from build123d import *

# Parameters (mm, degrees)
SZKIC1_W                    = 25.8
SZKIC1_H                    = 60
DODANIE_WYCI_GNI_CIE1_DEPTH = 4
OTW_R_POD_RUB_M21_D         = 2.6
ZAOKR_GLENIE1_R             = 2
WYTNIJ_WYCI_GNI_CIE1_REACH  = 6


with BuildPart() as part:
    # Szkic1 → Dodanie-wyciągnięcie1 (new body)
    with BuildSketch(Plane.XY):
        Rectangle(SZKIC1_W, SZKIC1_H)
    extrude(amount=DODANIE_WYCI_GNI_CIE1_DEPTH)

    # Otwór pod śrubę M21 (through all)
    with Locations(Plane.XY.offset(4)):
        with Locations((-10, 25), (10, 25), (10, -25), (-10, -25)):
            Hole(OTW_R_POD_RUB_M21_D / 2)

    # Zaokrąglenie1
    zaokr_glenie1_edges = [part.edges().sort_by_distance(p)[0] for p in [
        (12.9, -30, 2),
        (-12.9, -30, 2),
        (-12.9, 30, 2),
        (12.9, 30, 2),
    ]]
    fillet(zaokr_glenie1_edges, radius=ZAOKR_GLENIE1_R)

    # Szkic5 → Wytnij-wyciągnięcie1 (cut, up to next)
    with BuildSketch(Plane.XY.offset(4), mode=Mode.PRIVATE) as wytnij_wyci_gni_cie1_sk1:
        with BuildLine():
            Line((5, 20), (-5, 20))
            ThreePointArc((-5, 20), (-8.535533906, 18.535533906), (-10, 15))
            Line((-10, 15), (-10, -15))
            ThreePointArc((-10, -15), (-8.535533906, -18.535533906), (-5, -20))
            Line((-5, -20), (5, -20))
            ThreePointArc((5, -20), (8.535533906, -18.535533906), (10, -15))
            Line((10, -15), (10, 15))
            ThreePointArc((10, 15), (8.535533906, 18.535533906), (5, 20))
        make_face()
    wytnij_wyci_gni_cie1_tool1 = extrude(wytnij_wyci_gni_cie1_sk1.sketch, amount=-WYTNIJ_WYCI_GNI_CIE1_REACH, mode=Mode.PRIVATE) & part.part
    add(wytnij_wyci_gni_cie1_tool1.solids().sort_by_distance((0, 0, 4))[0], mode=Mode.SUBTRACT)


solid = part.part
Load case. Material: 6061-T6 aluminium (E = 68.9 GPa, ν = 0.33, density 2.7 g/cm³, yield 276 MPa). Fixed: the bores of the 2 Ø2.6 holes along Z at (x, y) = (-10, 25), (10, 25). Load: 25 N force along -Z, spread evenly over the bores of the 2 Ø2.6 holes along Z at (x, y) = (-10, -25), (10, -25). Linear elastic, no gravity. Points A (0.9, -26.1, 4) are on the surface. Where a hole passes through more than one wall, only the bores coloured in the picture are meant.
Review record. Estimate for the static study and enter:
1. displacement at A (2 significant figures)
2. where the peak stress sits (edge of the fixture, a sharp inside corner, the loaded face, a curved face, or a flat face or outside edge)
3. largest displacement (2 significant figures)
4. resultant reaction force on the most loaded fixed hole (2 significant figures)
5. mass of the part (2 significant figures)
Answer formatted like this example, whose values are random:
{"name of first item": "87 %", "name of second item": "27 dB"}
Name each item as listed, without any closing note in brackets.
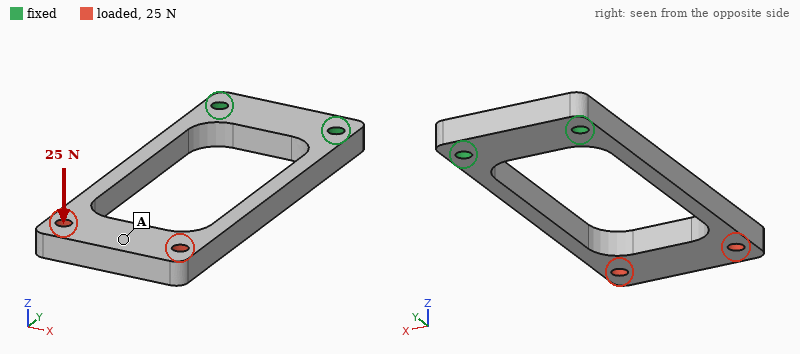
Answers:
{"displacement at A": "0.41 mm", "where the peak stress sits": "a curved face", "largest displacement": "0.46 mm", "resultant reaction force on the most loaded fixed hole": "13 N", "mass of the part": "8.0 g"}
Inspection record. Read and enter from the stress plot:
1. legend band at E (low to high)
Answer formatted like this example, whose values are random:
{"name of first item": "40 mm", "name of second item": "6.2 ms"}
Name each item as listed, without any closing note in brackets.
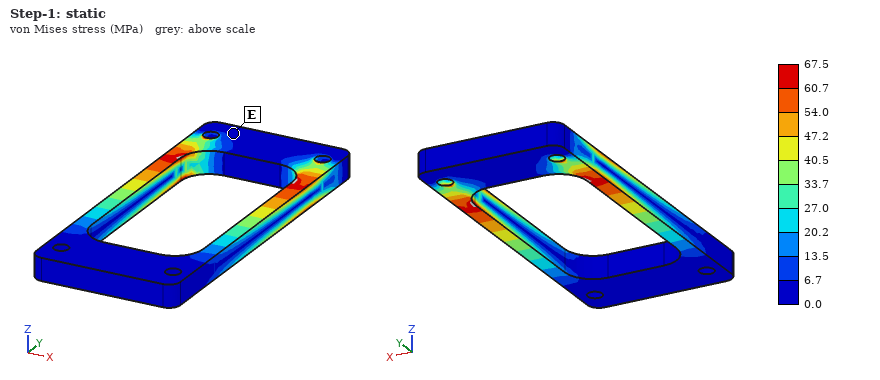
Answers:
{"legend band at E": "0.0 to 6.7 MPa"}
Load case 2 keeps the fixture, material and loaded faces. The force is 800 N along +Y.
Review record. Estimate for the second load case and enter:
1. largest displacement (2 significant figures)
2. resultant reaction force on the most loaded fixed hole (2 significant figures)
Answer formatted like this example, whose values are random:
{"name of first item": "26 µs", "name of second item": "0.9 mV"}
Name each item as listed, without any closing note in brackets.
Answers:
{"largest displacement": "26 µm", "resultant reaction force on the most loaded fixed hole": "400 N"}
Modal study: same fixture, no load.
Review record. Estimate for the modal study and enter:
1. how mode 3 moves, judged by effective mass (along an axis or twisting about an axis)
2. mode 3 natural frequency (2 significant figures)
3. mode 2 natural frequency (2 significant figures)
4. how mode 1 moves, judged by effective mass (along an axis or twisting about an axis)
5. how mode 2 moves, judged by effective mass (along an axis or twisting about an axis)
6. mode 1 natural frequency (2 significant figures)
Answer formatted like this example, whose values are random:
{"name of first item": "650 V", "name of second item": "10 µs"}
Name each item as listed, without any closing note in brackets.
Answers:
{"how mode 3 moves, judged by effective mass": "twisting about Y", "mode 3 natural frequency": "2400 Hz", "mode 2 natural frequency": "1300 Hz", "how mode 1 moves, judged by effective mass": "along Z", "how mode 2 moves, judged by effective mass": "along X", "mode 1 natural frequency": "710 Hz"}
